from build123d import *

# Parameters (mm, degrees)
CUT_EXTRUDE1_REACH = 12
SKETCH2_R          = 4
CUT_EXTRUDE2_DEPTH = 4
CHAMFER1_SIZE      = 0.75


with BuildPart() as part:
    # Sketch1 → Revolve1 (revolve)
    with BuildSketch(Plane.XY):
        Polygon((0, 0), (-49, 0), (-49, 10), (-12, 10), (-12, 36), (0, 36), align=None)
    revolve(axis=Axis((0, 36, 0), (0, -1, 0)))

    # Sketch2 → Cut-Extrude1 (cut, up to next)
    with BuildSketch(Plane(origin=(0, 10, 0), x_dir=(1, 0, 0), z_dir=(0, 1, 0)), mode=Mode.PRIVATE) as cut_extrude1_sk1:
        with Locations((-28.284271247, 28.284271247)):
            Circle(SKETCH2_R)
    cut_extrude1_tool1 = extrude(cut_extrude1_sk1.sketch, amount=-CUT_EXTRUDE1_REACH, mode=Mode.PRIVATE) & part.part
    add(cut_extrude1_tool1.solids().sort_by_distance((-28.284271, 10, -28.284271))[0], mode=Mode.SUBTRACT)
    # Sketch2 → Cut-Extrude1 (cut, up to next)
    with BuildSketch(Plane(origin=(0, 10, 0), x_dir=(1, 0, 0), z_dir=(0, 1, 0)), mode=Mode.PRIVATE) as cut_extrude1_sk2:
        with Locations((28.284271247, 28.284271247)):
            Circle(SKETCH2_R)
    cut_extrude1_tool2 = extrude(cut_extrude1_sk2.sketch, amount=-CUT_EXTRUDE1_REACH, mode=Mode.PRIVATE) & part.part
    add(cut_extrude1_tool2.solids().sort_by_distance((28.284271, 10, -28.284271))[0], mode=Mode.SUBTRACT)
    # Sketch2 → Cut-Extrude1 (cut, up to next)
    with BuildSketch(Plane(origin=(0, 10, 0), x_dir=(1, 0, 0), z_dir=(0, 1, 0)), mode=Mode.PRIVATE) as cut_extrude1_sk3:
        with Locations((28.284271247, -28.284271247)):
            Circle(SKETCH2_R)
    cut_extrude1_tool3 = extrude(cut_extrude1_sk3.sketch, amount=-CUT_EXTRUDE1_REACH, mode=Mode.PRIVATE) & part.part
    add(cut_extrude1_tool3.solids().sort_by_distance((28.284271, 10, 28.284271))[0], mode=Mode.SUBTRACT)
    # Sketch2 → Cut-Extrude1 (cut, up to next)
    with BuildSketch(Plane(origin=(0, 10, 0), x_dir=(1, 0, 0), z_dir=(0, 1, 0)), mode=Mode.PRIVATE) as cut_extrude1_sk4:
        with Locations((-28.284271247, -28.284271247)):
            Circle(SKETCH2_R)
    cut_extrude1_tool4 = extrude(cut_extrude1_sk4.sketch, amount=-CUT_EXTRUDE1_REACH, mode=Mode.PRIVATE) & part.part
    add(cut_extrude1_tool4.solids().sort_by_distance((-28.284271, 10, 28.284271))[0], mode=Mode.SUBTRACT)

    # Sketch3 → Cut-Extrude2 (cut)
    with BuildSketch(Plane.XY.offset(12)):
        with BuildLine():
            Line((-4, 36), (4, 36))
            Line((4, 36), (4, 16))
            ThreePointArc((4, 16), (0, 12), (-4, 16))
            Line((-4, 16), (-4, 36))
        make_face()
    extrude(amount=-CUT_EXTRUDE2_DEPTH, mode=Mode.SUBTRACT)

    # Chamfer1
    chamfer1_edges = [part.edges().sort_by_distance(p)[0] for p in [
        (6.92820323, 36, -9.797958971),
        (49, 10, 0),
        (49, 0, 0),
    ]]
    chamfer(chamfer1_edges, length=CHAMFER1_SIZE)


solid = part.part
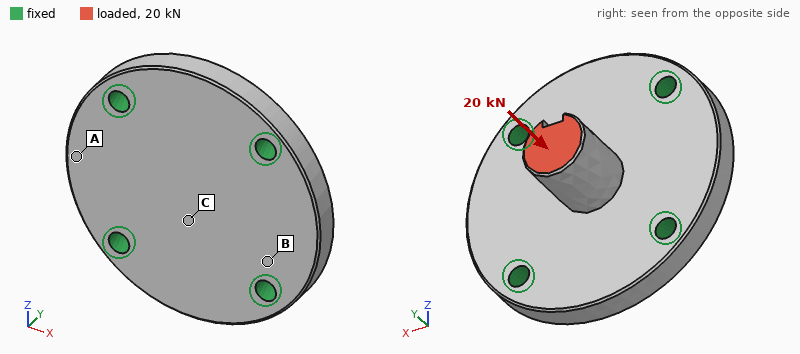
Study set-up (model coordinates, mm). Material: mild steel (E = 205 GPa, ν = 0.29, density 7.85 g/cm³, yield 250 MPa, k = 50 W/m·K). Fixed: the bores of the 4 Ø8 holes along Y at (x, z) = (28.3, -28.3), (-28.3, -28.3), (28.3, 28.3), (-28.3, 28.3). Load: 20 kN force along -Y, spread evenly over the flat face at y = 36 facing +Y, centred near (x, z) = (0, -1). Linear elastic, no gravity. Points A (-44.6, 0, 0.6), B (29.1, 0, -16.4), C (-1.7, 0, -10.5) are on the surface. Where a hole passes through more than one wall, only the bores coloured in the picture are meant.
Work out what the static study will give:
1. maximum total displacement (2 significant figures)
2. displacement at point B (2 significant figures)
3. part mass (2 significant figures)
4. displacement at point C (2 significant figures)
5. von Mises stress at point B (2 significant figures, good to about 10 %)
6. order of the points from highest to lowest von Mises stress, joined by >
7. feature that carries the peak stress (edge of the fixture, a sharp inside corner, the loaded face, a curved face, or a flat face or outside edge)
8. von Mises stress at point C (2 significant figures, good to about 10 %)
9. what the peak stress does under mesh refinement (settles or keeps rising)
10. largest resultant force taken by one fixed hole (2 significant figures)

37 µm
6.5 µm
660 g
30 µm
51 MPa
C > B > A
edge of the fixture
97 MPa
keeps rising
5.2 kN
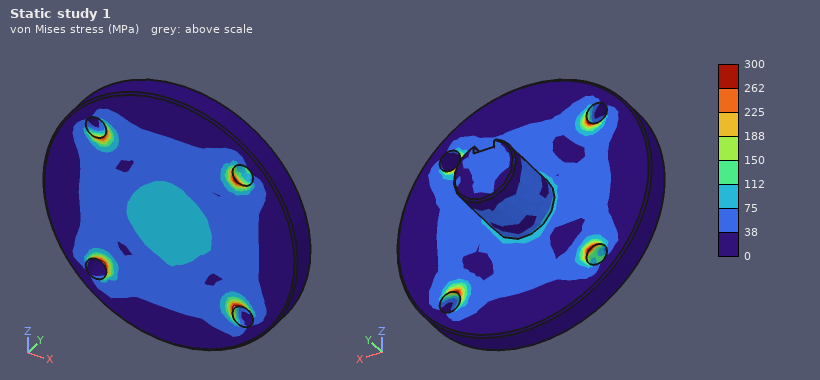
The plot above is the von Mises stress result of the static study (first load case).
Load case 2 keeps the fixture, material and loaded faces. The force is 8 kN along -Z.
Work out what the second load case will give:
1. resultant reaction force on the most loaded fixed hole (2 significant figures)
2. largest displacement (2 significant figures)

3.3 kN
63 µm
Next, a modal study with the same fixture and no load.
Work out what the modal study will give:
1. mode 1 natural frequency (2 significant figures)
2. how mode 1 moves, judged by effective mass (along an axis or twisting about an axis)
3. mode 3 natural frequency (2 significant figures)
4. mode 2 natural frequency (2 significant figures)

8900 Hz
along Y
9700 Hz
9700 Hz
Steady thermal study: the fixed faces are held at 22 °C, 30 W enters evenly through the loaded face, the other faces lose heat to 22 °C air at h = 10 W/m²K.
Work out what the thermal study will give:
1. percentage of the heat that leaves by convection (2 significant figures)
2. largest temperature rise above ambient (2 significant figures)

5.3 %
56 K
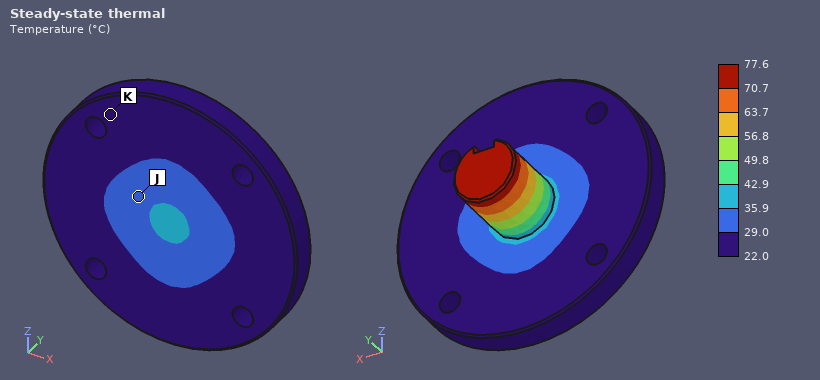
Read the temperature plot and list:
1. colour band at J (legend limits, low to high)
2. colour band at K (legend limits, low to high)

29.0 to 35.9 °C
22.0 to 29.0 °C
